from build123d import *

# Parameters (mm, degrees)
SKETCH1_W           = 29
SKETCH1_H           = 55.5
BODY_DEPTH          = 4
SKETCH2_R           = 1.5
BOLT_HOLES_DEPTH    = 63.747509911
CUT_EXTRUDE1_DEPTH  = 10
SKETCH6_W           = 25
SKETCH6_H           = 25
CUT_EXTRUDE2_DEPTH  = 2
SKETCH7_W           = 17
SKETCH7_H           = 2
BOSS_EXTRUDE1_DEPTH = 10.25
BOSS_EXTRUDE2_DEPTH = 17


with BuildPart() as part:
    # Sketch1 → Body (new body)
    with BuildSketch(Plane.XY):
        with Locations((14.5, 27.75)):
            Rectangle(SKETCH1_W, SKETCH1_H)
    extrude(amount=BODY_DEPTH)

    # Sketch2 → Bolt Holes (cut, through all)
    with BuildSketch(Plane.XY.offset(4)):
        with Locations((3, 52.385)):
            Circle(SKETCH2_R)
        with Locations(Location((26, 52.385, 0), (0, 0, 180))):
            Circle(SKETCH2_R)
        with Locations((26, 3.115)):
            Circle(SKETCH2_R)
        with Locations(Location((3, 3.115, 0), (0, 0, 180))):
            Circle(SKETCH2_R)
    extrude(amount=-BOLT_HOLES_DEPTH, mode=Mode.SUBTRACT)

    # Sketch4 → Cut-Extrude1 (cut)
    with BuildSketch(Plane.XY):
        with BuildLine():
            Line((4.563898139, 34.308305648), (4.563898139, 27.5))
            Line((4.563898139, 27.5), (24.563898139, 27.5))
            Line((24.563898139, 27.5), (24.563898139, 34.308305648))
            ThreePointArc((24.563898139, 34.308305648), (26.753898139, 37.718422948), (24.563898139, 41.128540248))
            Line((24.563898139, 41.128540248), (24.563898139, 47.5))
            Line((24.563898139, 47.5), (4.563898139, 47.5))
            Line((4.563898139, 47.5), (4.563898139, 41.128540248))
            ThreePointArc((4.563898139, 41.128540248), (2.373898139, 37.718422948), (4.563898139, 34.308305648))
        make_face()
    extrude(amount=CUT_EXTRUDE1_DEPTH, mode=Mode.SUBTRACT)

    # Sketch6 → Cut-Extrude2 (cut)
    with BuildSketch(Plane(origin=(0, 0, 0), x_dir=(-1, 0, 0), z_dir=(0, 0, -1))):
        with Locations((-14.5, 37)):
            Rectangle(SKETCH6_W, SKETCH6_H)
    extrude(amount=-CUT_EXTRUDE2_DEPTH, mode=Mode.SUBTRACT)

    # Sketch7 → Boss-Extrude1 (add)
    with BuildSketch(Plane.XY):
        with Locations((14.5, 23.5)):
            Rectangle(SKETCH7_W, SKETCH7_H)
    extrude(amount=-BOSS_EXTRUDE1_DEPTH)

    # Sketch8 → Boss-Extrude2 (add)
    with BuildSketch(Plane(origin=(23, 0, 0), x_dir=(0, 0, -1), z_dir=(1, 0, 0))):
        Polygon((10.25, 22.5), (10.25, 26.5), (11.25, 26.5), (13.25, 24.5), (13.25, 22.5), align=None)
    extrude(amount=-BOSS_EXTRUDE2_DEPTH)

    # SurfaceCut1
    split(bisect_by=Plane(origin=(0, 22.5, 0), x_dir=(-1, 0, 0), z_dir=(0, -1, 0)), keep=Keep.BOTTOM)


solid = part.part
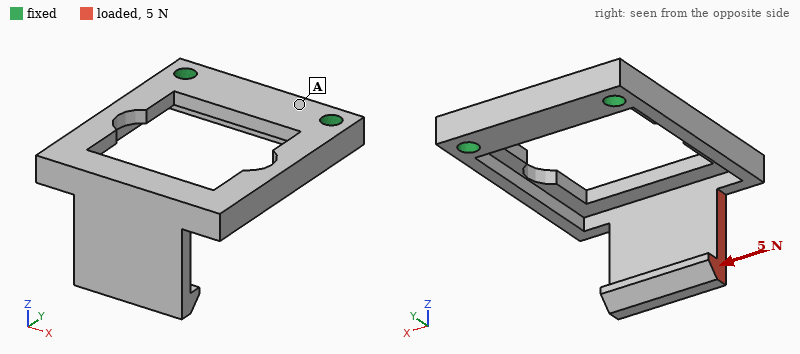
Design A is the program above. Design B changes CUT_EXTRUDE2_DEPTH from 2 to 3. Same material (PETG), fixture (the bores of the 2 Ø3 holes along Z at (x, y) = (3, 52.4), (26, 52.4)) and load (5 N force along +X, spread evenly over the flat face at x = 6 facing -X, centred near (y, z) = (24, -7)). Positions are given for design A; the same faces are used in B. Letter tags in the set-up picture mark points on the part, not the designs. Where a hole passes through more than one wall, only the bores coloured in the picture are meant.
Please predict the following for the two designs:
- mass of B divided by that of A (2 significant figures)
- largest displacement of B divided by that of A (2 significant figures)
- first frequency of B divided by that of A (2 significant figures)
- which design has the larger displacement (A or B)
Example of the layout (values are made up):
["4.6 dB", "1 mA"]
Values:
["0.91", "1.5", "1.00", "B"]
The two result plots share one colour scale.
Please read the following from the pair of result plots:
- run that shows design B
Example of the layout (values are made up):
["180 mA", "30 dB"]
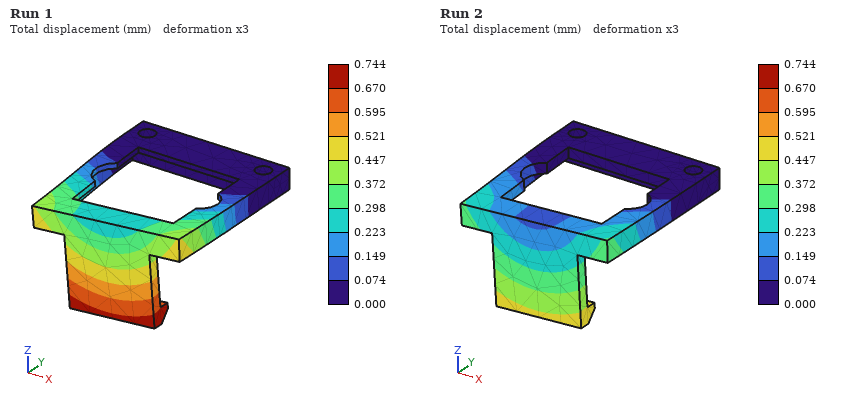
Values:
["Run 1"]
